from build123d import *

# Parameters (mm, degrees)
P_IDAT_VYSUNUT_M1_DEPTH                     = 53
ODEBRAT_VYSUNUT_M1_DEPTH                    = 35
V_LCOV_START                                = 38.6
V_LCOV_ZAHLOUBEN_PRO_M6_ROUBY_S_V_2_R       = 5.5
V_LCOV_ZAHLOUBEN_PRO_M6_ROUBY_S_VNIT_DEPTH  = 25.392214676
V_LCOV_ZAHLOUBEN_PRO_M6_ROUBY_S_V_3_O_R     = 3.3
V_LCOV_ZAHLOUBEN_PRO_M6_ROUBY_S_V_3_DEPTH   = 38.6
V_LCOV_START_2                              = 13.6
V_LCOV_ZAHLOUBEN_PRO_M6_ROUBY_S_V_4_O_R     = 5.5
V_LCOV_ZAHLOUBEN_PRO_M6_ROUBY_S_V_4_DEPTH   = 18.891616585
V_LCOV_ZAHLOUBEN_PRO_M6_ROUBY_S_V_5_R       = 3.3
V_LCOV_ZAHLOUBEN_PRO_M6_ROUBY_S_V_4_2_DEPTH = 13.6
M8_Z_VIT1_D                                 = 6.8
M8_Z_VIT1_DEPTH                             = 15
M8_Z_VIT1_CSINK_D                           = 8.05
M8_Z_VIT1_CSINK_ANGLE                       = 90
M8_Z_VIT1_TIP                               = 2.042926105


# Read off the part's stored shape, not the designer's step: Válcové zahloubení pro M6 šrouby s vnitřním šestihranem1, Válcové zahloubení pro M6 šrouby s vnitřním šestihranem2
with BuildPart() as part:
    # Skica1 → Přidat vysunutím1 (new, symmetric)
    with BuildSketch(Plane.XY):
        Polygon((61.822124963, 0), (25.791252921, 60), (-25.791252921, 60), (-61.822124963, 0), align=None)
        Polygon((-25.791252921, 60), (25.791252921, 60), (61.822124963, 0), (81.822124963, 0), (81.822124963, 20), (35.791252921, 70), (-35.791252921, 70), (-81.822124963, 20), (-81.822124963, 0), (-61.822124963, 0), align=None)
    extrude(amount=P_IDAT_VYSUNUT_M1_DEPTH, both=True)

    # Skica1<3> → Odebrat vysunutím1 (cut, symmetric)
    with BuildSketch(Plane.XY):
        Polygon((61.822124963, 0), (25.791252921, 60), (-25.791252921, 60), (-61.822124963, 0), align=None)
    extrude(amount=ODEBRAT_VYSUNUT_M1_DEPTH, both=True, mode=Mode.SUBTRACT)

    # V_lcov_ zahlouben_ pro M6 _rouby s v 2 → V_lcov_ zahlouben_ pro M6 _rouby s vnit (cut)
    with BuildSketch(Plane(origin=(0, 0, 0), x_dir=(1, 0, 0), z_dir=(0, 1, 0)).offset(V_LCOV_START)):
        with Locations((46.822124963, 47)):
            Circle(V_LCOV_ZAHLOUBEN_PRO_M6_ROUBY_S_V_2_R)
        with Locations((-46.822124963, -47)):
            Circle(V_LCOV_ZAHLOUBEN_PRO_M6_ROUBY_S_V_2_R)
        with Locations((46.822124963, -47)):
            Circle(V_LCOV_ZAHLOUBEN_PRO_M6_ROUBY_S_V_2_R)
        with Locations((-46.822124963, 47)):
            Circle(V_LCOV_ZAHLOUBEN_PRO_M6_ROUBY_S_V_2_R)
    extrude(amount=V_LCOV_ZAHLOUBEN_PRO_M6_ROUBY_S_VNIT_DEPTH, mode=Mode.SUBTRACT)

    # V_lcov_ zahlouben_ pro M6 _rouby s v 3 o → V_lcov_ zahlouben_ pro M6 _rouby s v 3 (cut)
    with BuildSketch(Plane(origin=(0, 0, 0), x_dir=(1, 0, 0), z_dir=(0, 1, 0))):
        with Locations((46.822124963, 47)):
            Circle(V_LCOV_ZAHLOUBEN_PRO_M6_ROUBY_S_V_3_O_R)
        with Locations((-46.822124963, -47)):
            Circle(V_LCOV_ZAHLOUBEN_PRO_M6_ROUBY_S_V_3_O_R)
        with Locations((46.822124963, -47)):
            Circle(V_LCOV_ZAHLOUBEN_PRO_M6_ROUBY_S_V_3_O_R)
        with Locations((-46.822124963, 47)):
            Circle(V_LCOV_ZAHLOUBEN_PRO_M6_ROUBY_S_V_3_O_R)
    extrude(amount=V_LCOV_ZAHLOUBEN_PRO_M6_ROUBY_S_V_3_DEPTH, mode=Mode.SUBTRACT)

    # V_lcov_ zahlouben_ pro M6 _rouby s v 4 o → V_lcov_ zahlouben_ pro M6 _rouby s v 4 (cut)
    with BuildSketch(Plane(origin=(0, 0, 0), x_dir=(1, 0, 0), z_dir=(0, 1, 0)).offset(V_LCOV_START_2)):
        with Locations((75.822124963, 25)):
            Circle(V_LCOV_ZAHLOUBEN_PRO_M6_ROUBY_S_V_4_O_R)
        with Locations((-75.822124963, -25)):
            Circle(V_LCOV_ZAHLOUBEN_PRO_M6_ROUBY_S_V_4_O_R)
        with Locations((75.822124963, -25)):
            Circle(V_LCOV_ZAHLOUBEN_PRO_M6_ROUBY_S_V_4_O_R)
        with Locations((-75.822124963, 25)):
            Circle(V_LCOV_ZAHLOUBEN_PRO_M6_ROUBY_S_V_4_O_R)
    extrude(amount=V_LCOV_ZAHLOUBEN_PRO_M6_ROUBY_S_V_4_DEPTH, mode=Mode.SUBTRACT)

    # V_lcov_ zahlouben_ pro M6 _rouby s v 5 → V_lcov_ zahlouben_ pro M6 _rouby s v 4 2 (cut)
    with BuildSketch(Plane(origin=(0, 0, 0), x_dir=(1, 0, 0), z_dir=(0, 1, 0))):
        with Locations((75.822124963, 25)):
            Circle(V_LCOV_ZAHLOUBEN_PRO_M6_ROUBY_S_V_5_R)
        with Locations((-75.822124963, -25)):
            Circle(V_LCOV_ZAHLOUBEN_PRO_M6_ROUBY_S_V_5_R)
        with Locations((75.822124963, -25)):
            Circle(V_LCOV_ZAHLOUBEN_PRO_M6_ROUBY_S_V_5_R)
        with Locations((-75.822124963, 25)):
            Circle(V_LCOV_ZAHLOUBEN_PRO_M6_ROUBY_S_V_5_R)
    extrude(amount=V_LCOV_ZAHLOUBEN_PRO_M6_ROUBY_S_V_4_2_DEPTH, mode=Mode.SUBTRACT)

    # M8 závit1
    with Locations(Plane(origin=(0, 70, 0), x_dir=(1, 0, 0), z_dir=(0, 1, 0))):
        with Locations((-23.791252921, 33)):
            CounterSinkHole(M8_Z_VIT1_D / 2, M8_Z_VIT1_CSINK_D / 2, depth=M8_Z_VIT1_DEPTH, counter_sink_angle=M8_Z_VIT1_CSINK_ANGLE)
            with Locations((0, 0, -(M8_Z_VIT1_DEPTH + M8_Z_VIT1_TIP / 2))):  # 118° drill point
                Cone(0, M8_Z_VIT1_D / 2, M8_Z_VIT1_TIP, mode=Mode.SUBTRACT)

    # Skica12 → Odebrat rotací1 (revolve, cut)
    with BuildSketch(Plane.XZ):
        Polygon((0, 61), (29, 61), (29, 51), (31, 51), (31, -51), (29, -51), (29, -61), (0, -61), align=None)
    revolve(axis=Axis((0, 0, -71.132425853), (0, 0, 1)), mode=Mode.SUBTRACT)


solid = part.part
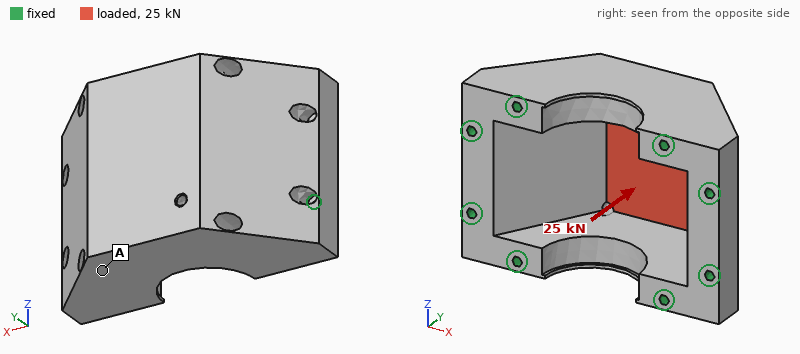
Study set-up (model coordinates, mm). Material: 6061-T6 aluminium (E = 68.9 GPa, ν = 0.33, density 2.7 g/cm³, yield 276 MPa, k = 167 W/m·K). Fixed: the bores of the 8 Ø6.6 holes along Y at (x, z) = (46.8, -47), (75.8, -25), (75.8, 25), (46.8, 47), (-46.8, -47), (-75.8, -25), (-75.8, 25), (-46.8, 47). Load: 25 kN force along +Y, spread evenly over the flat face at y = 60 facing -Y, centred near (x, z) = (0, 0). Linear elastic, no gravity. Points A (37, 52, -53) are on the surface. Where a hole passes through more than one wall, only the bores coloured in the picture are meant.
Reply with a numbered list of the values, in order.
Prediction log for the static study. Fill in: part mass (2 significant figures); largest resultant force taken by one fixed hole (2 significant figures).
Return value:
1. 1.4 kg
2. 6.0 kN
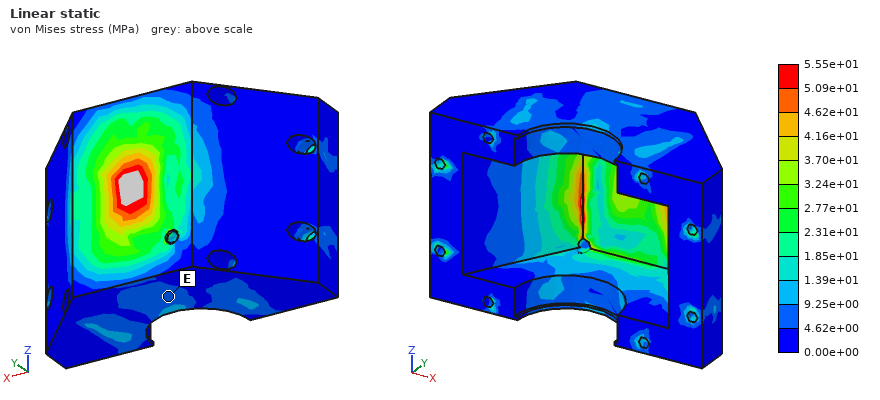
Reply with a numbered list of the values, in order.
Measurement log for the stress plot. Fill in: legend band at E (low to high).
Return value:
1. 4.62e+00 to 9.25e+00 MPa
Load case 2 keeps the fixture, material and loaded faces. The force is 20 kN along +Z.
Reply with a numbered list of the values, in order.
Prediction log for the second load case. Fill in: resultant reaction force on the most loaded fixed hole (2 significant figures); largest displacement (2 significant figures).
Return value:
1. 5.3 kN
2. 22 µm
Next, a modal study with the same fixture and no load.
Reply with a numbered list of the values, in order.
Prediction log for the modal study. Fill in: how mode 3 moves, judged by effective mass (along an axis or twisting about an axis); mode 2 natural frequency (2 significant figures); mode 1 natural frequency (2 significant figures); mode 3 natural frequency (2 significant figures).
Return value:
1. along Y
2. 9500 Hz
3. 9400 Hz
4. 11 kHz
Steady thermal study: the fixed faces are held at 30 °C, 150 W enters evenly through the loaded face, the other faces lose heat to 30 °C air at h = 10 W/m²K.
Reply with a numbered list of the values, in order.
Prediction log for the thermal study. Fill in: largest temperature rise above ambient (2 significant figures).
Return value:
1. 18 K
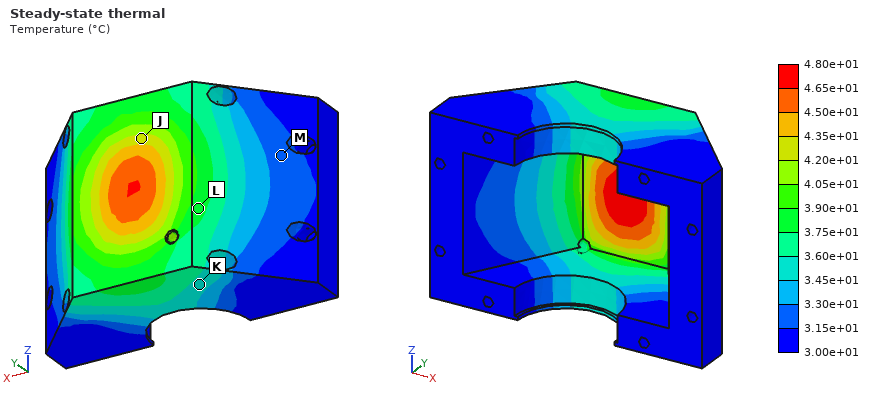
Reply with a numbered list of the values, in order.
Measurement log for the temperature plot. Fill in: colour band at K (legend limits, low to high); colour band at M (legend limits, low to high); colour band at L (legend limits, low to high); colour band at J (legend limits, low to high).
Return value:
1. 3.45e+01 to 3.60e+01 °C
2. 3.15e+01 to 3.30e+01 °C
3. 3.75e+01 to 3.90e+01 °C
4. 4.20e+01 to 4.35e+01 °C
